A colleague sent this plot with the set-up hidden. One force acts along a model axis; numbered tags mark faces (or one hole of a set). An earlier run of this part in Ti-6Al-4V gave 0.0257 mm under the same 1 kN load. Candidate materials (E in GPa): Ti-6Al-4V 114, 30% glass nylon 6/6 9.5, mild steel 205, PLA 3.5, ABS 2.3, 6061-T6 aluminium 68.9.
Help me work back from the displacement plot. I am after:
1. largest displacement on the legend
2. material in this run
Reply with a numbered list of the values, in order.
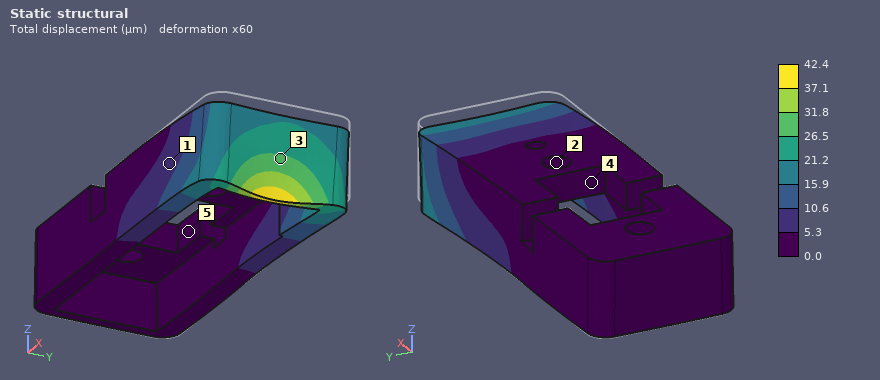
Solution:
1. 42.4 µm
2. 6061-T6 aluminium
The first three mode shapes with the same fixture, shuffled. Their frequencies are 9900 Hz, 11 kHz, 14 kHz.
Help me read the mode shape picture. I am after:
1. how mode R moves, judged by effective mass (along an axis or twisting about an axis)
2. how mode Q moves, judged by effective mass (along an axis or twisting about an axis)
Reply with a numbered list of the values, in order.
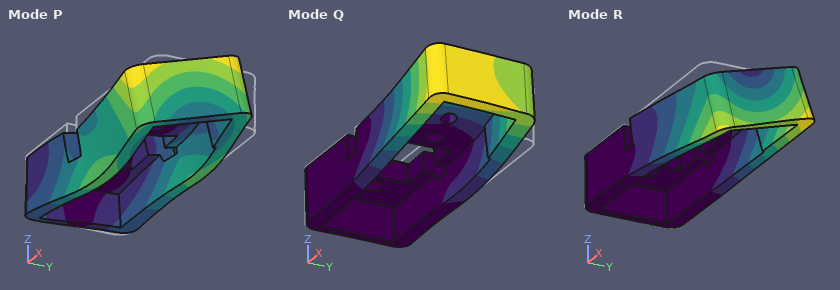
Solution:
1. along Y
2. along Z
